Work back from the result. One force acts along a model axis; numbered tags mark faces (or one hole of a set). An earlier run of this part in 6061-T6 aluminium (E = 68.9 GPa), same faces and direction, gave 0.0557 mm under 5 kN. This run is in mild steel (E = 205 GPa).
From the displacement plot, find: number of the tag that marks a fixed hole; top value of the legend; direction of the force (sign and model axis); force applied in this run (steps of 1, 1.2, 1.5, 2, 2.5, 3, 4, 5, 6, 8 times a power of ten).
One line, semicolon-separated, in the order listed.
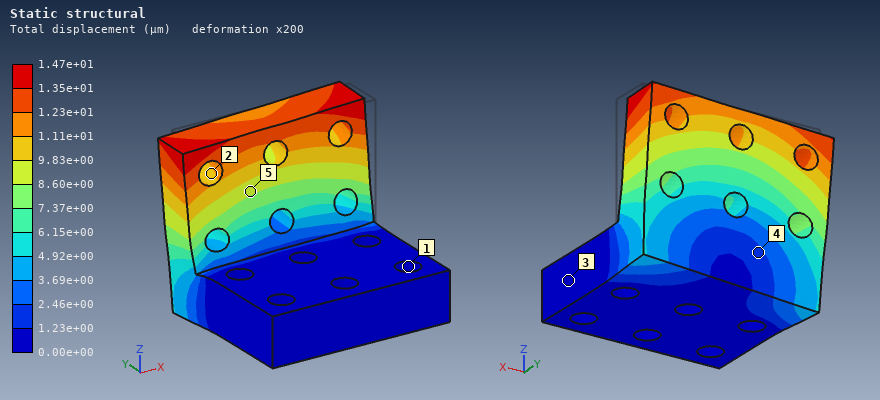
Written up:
1; 1.47e+01 µm; -X; 4 kN
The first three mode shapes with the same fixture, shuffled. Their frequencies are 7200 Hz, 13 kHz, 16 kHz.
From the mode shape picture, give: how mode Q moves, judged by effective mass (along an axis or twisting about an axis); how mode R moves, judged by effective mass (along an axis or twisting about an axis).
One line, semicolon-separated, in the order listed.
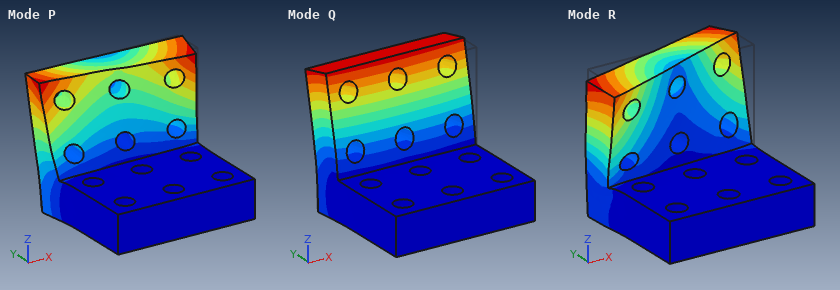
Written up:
along Y; along X
